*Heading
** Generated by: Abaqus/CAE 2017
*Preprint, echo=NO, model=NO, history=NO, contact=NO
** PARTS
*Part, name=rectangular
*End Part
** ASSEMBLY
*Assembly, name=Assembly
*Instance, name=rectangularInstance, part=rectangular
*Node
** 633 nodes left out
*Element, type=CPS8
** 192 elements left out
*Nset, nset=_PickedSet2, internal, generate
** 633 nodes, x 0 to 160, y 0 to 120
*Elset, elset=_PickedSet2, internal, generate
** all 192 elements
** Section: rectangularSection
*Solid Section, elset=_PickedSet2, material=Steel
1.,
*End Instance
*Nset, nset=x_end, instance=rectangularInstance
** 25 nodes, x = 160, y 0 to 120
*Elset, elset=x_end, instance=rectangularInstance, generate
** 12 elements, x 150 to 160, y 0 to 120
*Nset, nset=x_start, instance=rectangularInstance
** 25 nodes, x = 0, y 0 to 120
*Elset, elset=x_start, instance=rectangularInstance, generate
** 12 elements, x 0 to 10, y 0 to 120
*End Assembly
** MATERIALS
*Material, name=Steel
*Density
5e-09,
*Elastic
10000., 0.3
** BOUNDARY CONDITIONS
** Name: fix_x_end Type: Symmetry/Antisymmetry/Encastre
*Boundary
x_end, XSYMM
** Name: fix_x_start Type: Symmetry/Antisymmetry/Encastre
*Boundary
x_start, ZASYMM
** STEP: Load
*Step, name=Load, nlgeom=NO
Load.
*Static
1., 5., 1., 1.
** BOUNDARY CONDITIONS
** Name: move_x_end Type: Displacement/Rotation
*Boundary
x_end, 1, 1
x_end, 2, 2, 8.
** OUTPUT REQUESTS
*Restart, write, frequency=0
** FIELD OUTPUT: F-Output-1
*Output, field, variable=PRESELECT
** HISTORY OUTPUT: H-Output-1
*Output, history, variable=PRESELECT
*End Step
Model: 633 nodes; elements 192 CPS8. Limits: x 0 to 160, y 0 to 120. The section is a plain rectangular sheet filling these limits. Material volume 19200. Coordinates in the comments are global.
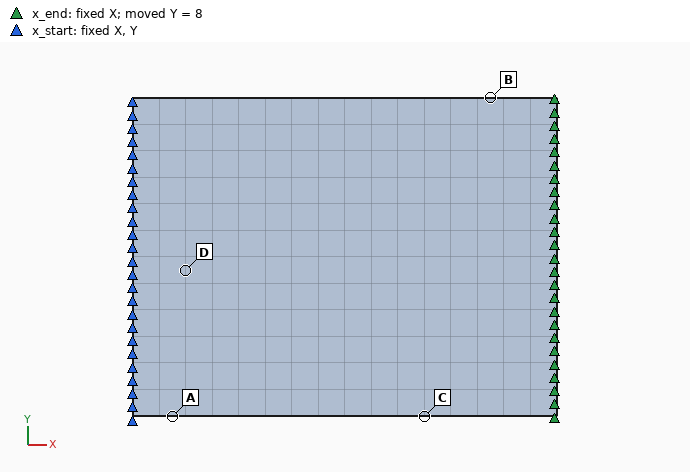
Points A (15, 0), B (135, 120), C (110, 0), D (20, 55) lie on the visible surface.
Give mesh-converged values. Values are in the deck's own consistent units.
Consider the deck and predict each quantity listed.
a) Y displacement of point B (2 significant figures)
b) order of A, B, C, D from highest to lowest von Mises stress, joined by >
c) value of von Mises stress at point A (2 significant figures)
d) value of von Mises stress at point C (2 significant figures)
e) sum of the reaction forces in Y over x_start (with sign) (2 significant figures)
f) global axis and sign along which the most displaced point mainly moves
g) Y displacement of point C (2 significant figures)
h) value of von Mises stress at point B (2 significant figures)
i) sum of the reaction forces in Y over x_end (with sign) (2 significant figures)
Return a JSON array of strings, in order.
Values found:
["6.9", "A > B > D > C", "380", "160", "-13000", "+Y", "5.7", "300", "13000"]
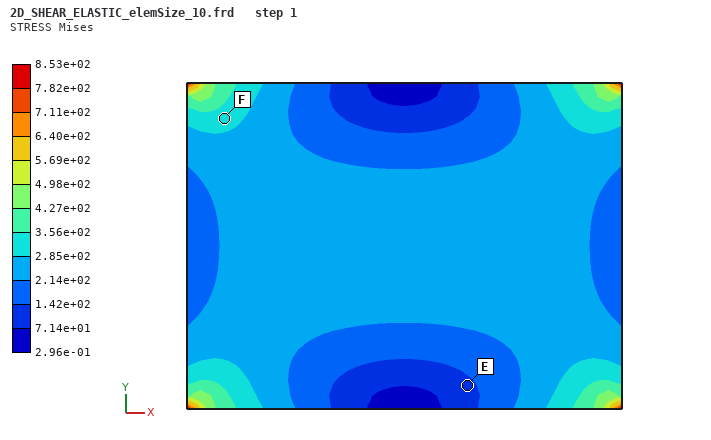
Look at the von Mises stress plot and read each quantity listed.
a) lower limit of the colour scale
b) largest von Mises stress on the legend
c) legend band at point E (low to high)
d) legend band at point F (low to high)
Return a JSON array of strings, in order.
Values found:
["2.96e-01", "8.53e+02", "7.14e+01 to 1.42e+02", "2.85e+02 to 3.56e+02"]
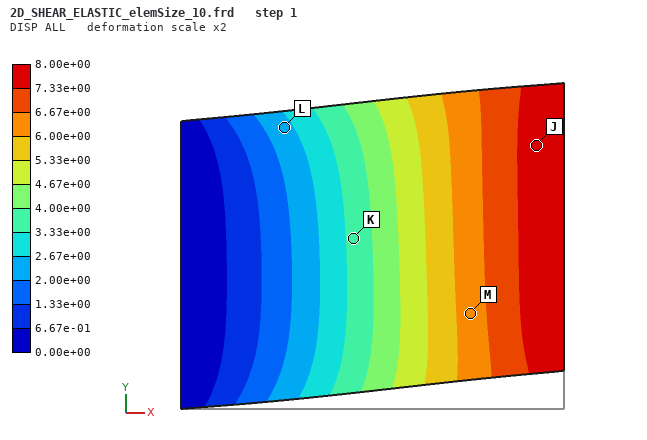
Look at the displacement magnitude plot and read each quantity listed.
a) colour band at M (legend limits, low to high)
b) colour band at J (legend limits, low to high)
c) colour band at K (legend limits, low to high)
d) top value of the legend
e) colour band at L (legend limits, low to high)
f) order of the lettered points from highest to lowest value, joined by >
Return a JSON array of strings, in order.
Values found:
["6.00e+00 to 6.67e+00", "7.33e+00 to 8.00e+00", "3.33e+00 to 4.00e+00", "8.00e+00", "2.00e+00 to 2.67e+00", "J > M > K > L"]
